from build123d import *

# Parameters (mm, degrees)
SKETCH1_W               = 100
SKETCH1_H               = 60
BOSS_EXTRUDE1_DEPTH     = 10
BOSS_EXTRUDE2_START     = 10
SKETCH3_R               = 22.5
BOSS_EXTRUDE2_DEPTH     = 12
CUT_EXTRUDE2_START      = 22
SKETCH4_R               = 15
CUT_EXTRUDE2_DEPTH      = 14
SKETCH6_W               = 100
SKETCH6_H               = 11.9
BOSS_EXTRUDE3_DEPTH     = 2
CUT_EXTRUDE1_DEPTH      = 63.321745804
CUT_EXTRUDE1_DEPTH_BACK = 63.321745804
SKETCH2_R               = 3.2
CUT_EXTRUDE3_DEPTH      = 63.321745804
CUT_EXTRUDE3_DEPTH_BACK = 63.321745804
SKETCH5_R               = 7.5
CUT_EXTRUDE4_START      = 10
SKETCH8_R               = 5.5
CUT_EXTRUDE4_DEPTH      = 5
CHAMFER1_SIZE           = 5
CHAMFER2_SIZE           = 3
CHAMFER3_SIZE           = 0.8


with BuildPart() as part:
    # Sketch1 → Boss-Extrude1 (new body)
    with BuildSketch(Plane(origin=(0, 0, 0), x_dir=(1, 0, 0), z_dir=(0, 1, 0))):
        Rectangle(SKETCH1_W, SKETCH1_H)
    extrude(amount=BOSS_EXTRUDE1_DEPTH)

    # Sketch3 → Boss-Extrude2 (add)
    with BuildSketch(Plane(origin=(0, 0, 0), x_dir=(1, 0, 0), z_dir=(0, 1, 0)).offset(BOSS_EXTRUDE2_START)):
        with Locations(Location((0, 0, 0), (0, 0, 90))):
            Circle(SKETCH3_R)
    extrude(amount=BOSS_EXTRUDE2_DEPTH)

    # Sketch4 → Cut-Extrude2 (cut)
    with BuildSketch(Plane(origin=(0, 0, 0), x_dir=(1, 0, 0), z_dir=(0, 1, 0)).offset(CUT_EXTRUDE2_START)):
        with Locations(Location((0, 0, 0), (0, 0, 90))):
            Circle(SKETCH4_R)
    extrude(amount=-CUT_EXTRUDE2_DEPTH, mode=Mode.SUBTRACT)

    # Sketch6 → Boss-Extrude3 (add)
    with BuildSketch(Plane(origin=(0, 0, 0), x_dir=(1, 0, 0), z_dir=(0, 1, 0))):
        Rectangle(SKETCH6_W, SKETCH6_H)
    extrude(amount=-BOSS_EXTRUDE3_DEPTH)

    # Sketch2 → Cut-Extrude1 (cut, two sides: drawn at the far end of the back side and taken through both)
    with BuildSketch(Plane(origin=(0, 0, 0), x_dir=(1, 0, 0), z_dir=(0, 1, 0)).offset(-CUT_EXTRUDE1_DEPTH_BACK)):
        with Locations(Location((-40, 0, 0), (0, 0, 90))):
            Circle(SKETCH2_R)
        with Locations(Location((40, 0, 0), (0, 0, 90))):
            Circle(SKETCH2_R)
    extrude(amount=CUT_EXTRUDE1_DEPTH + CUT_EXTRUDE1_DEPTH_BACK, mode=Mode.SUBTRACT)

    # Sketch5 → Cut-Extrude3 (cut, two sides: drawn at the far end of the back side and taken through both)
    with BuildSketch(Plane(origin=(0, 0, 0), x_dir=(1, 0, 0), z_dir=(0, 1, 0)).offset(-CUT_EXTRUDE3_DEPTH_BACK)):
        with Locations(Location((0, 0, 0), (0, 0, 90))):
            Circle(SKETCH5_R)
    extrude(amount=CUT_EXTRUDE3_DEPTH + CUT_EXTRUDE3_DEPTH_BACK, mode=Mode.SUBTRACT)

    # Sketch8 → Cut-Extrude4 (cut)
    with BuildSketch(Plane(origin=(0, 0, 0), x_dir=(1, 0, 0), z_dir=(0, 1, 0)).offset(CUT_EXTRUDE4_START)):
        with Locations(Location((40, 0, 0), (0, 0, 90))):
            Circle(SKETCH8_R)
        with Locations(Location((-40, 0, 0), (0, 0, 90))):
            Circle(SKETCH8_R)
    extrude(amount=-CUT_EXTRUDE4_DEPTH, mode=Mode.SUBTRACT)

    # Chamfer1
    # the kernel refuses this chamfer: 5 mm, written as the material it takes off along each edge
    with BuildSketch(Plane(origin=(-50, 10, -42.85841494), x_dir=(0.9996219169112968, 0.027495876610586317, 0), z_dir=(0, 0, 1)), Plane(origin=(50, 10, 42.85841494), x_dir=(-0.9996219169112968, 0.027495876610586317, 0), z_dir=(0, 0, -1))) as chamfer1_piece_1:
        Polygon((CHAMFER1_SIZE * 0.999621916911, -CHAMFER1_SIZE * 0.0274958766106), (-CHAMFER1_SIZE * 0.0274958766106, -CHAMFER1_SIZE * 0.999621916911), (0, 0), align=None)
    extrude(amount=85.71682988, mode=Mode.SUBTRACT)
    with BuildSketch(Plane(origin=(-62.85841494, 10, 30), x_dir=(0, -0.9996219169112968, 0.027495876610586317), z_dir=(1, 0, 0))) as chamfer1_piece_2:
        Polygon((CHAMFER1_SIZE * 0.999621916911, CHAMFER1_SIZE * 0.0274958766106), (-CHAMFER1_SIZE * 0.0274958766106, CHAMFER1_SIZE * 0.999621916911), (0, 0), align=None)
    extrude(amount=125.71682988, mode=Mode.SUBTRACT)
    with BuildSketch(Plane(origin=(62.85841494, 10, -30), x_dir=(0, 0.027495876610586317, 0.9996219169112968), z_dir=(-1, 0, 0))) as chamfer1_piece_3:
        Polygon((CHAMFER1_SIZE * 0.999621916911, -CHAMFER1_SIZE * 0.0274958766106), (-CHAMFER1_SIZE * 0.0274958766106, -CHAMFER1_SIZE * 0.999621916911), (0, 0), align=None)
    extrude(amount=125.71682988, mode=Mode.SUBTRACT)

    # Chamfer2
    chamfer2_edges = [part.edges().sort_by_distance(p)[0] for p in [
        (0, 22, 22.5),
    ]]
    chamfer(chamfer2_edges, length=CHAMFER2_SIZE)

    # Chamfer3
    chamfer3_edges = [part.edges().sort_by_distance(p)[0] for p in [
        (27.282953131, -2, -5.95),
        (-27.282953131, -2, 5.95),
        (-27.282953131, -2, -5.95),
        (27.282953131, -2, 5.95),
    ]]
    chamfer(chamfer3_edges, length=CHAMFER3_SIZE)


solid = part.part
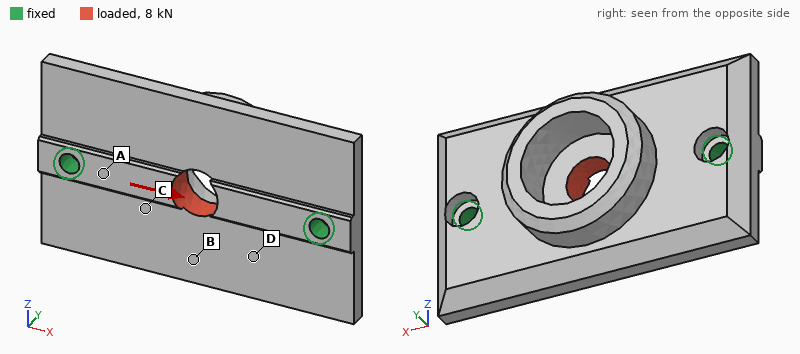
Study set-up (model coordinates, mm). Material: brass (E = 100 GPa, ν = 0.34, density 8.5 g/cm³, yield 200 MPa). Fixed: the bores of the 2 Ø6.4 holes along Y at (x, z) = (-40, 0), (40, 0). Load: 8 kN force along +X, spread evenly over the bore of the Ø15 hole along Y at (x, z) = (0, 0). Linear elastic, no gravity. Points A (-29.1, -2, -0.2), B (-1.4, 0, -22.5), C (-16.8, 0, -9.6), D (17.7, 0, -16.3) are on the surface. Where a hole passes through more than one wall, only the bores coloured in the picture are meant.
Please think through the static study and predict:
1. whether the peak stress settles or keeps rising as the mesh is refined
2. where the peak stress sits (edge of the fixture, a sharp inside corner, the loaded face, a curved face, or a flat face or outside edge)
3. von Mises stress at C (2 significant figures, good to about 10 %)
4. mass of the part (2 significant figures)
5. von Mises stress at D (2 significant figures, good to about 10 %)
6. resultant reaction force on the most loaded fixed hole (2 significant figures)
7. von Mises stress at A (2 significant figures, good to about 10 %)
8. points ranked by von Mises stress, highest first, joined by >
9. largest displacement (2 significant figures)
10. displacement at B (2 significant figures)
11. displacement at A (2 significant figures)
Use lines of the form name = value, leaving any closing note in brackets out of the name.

whether the peak stress settles or keeps rising as the mesh is refined = keeps rising
where the peak stress sits = edge of the fixture
von Mises stress at C = 15 MPa
mass of the part = 540 g
von Mises stress at D = 8.6 MPa
resultant reaction force on the most loaded fixed hole = 4.0 kN
von Mises stress at A = 30 MPa
points ranked by von Mises stress, highest first, joined by > = A > C > D > B
largest displacement = 7.8 µm
displacement at B = 5.0 µm
displacement at A = 2.3 µm
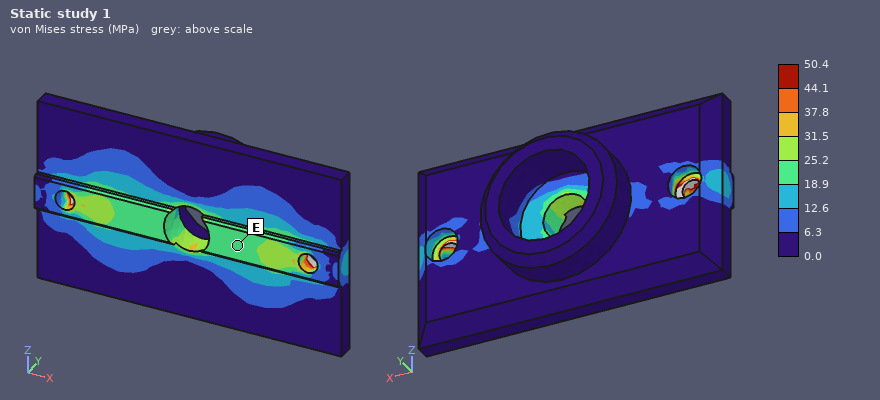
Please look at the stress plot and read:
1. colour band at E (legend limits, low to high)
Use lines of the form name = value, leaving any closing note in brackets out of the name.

colour band at E = 18.9 to 25.2 MPa
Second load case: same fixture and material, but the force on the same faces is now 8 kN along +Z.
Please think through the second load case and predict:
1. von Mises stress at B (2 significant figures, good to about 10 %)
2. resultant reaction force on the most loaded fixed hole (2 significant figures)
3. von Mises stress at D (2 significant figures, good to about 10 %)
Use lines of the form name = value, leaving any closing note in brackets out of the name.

von Mises stress at B = 18 MPa
resultant reaction force on the most loaded fixed hole = 4.0 kN
von Mises stress at D = 17 MPa
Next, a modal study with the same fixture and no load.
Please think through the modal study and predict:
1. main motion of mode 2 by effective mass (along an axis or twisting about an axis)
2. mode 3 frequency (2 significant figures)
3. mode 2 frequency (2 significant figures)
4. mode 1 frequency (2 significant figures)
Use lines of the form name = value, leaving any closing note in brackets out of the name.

main motion of mode 2 by effective mass = along Y
mode 3 frequency = 5700 Hz
mode 2 frequency = 3700 Hz
mode 1 frequency = 2300 Hz
